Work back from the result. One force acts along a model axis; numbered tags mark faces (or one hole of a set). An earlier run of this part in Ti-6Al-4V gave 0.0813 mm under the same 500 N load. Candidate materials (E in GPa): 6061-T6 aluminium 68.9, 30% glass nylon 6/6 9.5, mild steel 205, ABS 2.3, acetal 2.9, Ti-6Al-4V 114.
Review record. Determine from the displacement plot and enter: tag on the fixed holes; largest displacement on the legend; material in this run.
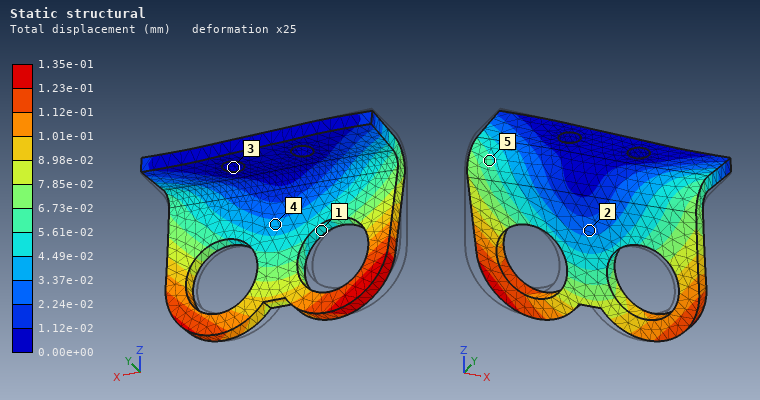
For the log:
3
1.35e-01 mm
6061-T6 aluminium
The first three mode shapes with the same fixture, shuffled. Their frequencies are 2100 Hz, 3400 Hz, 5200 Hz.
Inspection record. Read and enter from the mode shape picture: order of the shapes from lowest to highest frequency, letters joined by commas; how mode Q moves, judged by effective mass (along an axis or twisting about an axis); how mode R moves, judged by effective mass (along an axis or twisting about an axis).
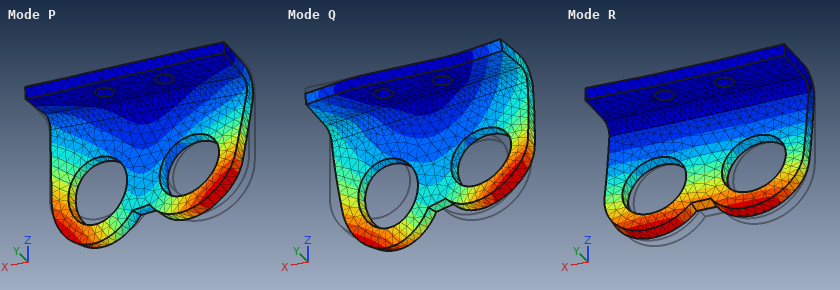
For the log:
R, P, Q
along X
along Y
